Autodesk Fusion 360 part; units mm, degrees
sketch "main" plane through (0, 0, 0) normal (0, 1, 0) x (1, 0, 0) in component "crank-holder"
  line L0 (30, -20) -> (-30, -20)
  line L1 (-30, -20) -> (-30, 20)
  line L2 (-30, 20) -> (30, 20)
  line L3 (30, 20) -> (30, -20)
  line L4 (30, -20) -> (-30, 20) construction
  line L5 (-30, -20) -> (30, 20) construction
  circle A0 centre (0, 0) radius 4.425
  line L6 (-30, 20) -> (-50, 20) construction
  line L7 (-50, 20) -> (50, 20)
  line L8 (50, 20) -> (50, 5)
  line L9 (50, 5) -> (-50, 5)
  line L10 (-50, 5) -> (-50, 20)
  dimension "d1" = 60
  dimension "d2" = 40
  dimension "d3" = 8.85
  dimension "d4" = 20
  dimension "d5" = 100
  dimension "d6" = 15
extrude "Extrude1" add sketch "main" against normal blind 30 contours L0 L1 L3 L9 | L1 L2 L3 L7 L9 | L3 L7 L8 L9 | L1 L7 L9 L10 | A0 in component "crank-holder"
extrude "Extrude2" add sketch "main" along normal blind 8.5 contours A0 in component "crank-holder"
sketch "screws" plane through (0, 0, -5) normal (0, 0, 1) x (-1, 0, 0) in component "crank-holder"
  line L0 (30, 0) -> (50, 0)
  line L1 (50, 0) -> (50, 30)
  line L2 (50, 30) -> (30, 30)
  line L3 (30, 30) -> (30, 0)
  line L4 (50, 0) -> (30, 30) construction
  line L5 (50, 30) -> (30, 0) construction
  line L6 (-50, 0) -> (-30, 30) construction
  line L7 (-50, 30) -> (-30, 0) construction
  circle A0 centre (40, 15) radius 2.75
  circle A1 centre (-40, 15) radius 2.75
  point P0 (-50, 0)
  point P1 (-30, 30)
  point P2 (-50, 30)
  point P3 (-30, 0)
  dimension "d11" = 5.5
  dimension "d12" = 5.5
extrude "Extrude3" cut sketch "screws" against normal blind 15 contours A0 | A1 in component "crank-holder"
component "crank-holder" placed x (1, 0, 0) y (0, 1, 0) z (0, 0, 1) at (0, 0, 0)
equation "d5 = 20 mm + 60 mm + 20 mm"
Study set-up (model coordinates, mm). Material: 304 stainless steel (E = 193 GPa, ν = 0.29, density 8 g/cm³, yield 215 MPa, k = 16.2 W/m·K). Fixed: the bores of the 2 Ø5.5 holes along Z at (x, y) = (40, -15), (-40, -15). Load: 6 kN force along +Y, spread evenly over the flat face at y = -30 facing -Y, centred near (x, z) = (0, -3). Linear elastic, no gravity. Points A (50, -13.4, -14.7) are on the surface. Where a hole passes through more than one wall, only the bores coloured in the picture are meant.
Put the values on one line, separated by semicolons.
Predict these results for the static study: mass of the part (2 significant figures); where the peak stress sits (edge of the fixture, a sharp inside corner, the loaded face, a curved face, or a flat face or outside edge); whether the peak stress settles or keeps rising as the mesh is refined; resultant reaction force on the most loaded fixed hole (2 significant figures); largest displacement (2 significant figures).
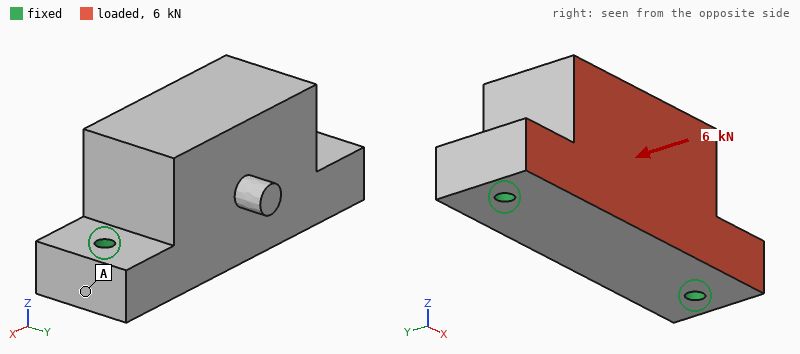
720 g; edge of the fixture; keeps rising; 3.0 kN; 15 µm
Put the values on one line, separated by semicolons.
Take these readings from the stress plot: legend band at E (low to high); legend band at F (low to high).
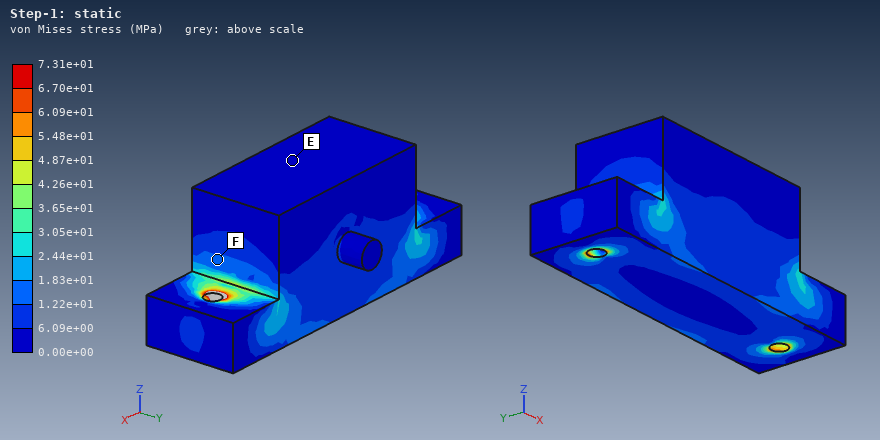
0.00e+00 to 6.09e+00 MPa; 1.22e+01 to 1.83e+01 MPa
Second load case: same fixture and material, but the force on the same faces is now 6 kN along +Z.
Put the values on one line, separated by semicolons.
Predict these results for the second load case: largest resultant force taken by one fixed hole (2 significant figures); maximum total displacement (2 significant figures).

3.1 kN; 17 µm
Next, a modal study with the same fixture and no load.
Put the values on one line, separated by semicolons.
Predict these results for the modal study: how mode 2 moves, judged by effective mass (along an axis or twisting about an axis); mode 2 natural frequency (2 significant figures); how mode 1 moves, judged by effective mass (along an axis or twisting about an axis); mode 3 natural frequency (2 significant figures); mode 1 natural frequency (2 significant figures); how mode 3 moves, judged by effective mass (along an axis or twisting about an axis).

along Z; 8700 Hz; along Y; 11 kHz; 4400 Hz; along Y
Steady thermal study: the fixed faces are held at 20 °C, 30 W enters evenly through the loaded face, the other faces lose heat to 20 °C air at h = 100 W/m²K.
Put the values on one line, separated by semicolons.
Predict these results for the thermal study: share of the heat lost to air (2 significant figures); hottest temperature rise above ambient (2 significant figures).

50 %; 27 K
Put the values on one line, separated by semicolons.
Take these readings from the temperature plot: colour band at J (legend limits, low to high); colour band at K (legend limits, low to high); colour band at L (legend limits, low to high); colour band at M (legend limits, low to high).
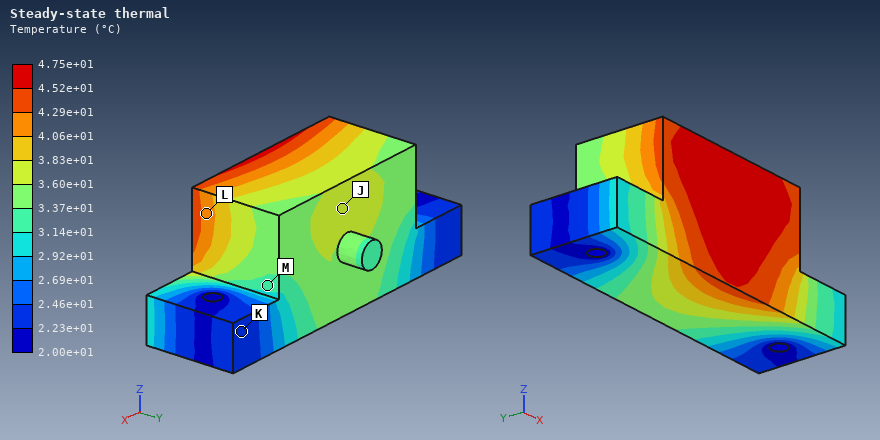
3.60e+01 to 3.83e+01 °C; 2.23e+01 to 2.46e+01 °C; 4.06e+01 to 4.29e+01 °C; 3.14e+01 to 3.37e+01 °C
